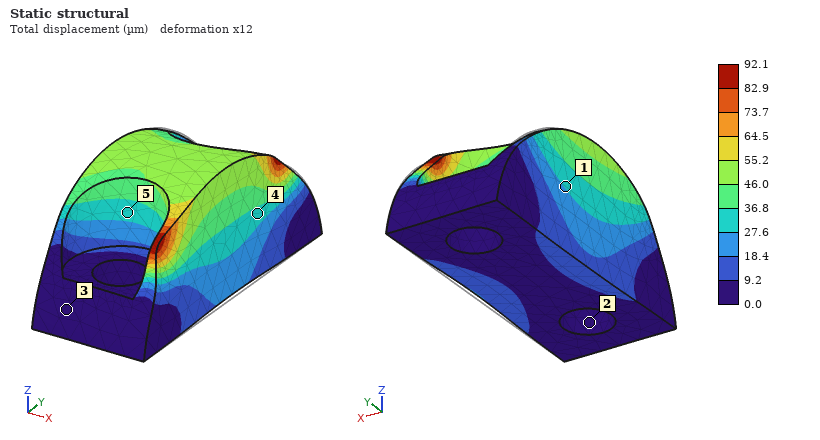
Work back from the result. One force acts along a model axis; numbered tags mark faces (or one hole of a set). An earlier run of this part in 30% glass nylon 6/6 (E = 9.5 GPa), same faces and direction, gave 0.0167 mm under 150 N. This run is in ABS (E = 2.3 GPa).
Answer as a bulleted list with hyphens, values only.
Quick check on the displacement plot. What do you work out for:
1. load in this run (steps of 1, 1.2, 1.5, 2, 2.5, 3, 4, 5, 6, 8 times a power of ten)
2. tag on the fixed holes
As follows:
- 200 N
- 2
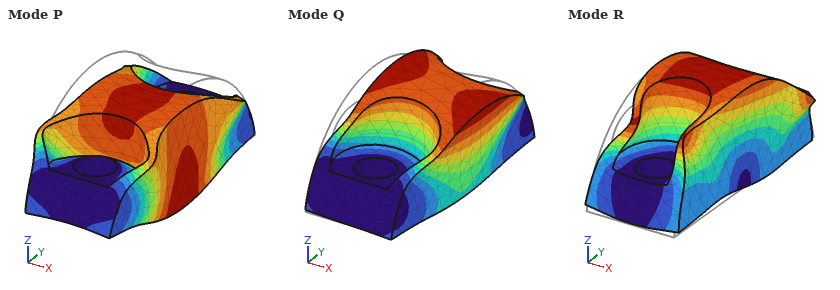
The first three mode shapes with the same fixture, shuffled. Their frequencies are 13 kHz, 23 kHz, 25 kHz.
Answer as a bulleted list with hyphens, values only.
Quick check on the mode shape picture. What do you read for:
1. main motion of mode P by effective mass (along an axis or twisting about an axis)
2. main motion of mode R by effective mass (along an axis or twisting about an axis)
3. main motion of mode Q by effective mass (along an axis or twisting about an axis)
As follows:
- along Z
- along Y
- along X
